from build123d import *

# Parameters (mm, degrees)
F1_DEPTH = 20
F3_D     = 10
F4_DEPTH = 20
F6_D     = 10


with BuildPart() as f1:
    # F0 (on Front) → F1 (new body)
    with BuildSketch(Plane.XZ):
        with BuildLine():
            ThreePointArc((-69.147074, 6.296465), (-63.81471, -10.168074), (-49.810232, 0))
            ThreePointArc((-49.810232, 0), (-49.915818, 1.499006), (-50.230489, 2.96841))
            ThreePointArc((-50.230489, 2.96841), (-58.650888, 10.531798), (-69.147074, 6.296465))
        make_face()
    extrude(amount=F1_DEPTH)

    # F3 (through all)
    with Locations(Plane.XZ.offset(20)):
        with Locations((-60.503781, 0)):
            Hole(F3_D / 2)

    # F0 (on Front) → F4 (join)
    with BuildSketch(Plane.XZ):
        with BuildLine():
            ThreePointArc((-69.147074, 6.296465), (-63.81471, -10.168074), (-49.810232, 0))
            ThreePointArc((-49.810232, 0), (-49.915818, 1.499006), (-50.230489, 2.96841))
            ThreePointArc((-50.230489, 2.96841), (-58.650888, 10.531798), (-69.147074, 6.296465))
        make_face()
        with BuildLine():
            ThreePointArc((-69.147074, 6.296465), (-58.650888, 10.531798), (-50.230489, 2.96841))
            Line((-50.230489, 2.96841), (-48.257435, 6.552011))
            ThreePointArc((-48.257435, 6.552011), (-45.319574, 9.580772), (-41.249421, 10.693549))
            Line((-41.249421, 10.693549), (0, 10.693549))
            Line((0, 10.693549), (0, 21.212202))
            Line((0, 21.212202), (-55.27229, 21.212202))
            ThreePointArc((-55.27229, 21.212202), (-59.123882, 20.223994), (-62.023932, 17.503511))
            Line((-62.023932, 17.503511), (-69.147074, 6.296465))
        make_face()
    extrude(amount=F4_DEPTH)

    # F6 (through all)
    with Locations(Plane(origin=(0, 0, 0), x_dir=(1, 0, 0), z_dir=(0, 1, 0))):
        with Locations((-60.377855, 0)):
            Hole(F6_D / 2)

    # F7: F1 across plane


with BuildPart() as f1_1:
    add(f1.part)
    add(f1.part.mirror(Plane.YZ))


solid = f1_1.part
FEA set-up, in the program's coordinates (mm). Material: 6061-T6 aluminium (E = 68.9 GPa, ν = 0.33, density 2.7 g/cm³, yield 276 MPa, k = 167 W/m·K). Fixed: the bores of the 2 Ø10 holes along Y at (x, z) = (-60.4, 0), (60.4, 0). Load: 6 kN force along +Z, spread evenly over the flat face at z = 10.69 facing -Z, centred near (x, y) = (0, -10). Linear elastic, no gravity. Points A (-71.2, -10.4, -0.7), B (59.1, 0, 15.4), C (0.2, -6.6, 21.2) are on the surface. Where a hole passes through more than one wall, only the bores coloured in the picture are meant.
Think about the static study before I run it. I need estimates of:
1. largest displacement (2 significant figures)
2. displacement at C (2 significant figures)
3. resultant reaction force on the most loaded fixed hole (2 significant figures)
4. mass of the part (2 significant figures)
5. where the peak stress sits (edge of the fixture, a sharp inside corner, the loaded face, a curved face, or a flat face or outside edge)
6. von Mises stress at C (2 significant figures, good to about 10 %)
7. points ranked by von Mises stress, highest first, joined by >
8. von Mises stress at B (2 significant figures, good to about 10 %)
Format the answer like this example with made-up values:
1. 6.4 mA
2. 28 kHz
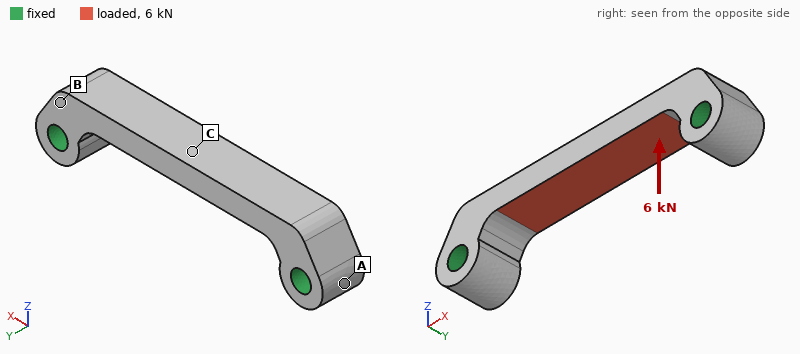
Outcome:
1. 0.18 mm
2. 0.18 mm
3. 4.3 kN
4. 110 g
5. a curved face
6. 100 MPa
7. C > B > A
8. 29 MPa
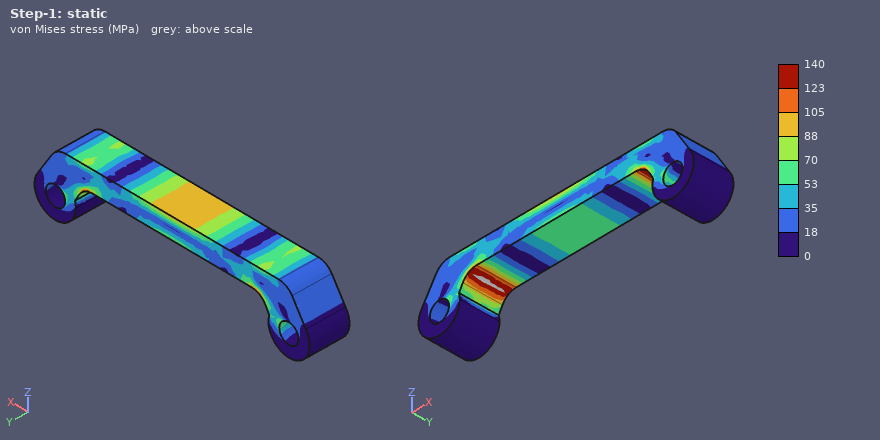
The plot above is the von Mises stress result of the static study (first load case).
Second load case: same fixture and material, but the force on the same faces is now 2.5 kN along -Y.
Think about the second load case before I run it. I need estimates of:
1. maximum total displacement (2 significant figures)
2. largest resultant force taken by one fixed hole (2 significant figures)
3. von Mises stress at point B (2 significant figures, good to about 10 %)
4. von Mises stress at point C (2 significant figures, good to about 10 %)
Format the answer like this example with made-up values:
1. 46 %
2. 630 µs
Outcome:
1. 55 µm
2. 1.3 kN
3. 15 MPa
4. 10 MPa
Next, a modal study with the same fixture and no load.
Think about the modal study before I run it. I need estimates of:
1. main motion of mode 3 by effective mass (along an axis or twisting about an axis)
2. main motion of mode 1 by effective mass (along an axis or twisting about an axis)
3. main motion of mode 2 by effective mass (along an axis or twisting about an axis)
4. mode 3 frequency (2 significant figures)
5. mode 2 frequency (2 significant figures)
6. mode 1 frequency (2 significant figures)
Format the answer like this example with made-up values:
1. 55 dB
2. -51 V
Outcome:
1. along X
2. along Z
3. along Y
4. 9900 Hz
5. 5900 Hz
6. 4700 Hz
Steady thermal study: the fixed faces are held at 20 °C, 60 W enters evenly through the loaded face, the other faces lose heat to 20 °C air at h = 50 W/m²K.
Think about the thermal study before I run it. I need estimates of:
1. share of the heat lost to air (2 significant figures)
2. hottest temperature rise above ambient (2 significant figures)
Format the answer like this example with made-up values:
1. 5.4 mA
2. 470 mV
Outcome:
1. 8.4 %
2. 30 K
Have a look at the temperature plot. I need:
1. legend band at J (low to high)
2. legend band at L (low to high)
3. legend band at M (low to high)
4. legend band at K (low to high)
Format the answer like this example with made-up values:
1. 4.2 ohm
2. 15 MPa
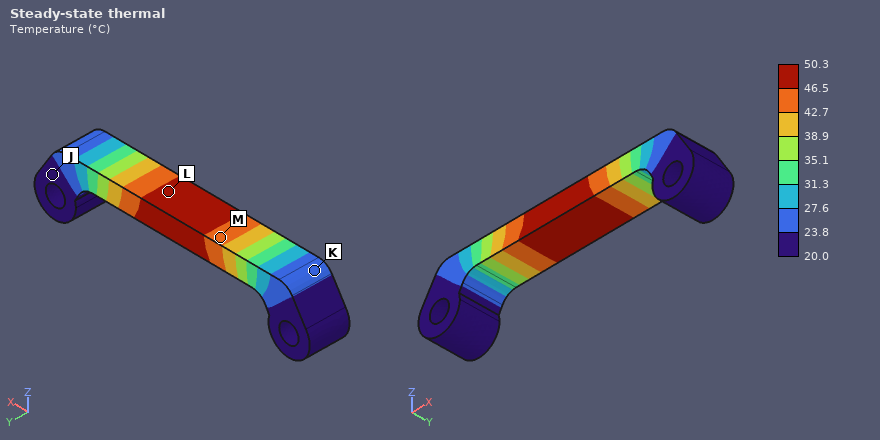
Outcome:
1. 20.0 to 23.8 °C
2. 46.5 to 50.3 °C
3. 42.7 to 46.5 °C
4. 23.8 to 27.6 °C
